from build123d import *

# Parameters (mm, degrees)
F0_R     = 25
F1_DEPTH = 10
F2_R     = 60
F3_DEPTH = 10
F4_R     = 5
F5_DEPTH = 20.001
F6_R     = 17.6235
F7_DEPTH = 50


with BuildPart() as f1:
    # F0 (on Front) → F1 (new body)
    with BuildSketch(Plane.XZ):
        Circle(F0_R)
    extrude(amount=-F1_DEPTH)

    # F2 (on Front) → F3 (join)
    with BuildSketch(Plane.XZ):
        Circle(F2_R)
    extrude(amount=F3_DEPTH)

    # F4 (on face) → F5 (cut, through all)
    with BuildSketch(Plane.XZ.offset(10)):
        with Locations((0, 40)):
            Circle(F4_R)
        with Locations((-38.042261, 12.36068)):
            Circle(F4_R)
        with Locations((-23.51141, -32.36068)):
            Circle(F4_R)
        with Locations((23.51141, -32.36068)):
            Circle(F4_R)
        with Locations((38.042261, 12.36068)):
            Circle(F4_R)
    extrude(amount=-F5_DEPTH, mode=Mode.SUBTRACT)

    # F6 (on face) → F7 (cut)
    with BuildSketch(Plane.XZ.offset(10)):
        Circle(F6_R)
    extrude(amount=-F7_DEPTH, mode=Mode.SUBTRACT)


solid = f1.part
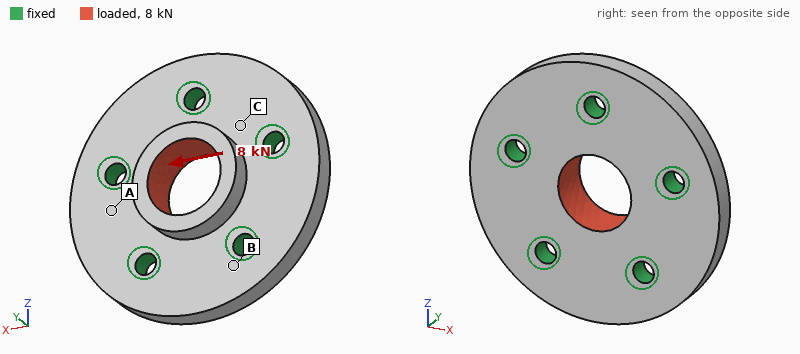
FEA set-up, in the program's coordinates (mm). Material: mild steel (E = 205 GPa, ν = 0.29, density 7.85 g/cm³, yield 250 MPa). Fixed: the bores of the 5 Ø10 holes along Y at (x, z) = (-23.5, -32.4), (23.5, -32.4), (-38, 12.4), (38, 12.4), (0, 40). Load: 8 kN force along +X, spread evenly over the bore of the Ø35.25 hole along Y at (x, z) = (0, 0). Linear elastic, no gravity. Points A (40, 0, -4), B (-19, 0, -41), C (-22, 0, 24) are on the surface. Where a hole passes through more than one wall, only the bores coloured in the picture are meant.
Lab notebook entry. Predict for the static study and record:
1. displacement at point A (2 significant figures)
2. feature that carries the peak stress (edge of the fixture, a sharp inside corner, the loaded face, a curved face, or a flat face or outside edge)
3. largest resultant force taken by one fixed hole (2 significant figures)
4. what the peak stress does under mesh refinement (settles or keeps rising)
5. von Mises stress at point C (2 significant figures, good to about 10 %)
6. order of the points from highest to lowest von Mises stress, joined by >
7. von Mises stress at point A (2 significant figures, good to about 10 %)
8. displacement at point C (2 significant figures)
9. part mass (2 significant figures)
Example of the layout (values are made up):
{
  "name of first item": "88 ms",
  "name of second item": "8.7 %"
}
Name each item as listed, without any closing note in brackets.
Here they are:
{
  "displacement at point A": "0.43 µm",
  "feature that carries the peak stress": "edge of the fixture",
  "largest resultant force taken by one fixed hole": "2.1 kN",
  "what the peak stress does under mesh refinement": "keeps rising",
  "von Mises stress at point C": "5.0 MPa",
  "order of the points from highest to lowest von Mises stress, joined by >": "C > A > B",
  "von Mises stress at point A": "2.8 MPa",
  "displacement at point C": "0.43 µm",
  "part mass": "860 g"
}
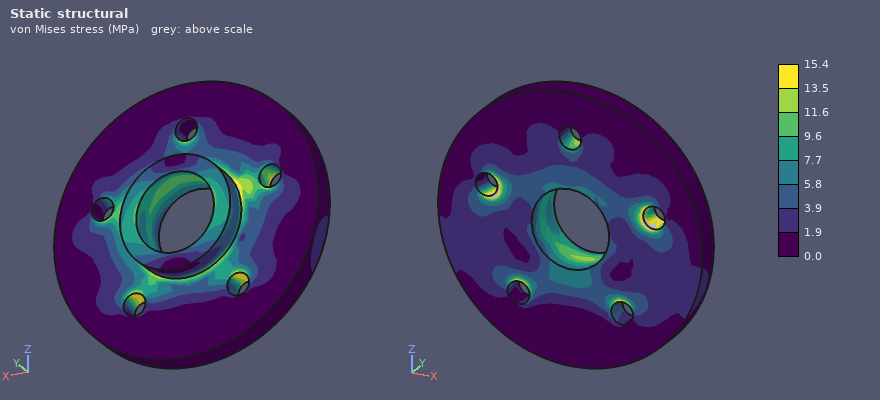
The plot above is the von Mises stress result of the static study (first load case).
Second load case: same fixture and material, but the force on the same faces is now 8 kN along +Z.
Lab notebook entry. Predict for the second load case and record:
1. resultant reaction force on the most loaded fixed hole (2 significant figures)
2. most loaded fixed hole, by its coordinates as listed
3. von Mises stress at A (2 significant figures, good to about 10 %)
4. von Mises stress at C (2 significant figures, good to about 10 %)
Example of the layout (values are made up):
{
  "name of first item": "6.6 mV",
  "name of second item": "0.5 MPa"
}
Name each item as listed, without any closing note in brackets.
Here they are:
{
  "resultant reaction force on the most loaded fixed hole": "2.2 kN",
  "most loaded fixed hole, by its coordinates as listed": "(0, 40)",
  "von Mises stress at A": "1.3 MPa",
  "von Mises stress at C": "4.4 MPa"
}
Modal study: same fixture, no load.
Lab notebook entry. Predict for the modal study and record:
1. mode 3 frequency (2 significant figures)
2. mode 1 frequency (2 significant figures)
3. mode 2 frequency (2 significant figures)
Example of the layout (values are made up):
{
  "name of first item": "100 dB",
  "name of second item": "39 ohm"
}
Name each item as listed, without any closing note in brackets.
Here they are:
{
  "mode 3 frequency": "12 kHz",
  "mode 1 frequency": "11 kHz",
  "mode 2 frequency": "11 kHz"
}
